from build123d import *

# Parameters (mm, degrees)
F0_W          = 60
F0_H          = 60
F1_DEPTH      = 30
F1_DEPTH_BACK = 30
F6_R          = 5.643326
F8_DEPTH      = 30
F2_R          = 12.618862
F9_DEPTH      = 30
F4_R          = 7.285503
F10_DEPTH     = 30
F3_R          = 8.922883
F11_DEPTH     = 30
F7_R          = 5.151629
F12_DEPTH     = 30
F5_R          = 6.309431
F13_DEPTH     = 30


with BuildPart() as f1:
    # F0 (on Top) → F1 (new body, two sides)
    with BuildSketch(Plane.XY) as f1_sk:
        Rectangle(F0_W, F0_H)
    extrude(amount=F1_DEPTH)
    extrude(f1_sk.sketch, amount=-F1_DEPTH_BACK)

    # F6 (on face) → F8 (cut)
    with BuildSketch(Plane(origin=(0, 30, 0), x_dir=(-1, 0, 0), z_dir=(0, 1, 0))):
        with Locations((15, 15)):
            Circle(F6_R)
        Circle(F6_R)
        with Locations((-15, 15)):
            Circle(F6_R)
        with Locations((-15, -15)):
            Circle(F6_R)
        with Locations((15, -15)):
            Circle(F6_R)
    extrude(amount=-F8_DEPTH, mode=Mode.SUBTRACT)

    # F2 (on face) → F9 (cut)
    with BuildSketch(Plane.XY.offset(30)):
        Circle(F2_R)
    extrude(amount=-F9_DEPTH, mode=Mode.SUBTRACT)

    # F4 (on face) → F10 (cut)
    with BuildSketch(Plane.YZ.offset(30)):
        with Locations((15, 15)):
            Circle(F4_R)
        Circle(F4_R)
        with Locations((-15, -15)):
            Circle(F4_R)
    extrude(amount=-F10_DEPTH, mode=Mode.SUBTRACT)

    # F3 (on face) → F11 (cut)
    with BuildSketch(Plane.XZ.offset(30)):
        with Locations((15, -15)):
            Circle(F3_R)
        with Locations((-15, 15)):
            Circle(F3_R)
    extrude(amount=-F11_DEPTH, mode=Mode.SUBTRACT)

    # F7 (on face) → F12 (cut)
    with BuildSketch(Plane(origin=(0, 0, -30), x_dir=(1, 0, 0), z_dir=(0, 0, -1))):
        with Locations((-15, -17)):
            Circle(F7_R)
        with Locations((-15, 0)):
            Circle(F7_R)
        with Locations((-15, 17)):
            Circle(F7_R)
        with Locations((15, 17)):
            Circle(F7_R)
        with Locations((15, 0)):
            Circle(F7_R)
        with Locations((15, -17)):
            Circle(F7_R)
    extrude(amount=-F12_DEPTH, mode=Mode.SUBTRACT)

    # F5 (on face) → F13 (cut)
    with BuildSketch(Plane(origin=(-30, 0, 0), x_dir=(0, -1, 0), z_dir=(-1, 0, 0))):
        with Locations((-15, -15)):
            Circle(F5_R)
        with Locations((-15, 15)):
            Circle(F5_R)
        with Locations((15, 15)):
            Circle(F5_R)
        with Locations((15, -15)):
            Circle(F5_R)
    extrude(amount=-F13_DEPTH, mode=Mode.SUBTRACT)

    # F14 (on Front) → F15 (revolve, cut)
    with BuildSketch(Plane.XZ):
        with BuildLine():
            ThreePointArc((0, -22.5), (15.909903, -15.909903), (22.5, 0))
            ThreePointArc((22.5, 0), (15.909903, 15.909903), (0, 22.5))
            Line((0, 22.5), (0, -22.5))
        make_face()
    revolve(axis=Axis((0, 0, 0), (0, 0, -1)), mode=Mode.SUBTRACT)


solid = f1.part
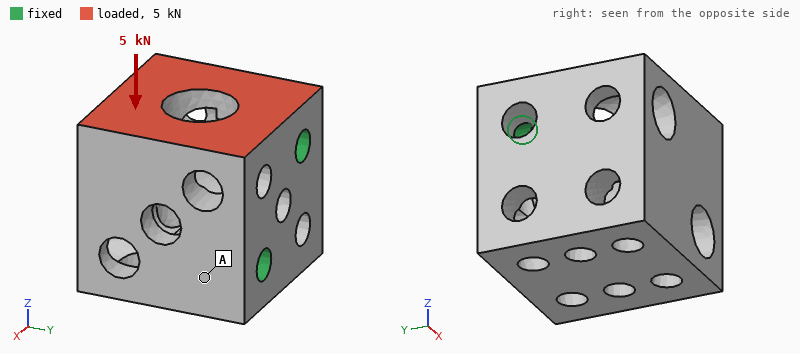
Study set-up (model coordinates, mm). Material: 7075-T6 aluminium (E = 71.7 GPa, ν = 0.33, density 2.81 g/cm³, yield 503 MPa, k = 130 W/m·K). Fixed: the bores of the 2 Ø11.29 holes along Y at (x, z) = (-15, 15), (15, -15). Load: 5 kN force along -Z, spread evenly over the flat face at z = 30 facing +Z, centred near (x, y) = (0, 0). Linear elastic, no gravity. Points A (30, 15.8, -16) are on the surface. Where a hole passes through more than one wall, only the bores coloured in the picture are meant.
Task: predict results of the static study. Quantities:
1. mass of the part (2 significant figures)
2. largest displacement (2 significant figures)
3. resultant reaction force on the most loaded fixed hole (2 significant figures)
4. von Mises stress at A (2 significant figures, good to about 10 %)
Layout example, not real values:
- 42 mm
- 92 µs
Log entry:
- 340 g
- 27 µm
- 2.8 kN
- 4.0 MPa
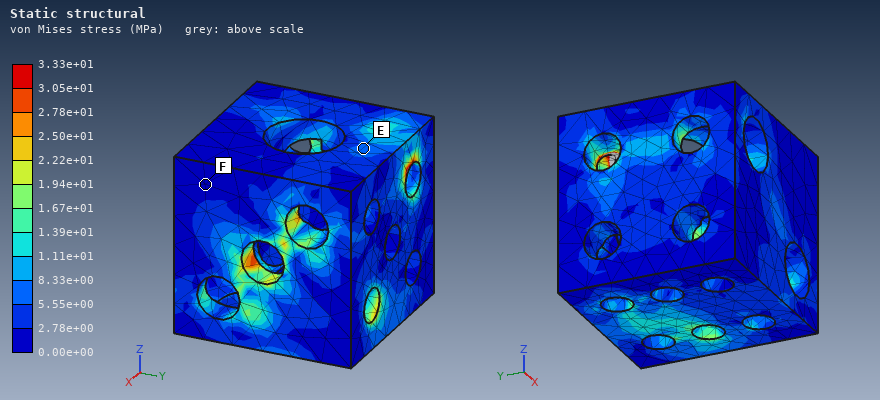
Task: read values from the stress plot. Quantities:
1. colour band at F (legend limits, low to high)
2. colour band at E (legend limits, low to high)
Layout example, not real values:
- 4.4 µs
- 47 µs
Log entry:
- 0.00e+00 to 2.78e+00 MPa
- 5.55e+00 to 8.33e+00 MPa
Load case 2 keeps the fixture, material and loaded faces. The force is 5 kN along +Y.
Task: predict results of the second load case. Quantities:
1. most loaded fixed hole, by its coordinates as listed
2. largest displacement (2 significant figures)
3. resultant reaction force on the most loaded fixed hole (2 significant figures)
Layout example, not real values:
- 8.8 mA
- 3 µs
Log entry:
- (-15, 15)
- 34 µm
- 4.2 kN
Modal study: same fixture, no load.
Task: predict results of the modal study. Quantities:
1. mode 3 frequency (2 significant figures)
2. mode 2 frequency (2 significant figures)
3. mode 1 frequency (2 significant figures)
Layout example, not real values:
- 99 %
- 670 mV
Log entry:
- 9100 Hz
- 6000 Hz
- 3700 Hz
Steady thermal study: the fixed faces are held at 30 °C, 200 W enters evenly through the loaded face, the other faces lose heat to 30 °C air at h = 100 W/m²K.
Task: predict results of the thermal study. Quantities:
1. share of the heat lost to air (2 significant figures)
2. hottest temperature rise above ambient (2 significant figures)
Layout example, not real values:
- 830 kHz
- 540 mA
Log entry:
- 24 %
- 45 K
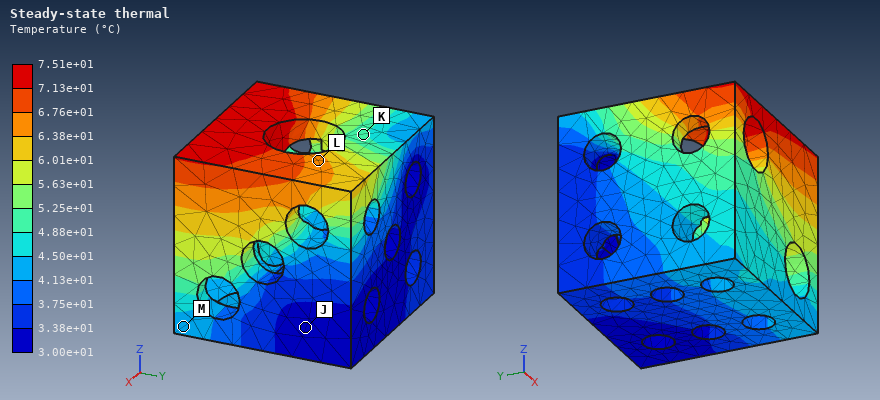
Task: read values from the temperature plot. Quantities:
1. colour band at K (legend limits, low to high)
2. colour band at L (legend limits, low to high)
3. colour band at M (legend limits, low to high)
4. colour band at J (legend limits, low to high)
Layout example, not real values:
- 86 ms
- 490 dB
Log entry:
- 4.88e+01 to 5.25e+01 °C
- 6.38e+01 to 6.76e+01 °C
- 4.13e+01 to 4.50e+01 °C
- 3.00e+01 to 3.38e+01 °C
